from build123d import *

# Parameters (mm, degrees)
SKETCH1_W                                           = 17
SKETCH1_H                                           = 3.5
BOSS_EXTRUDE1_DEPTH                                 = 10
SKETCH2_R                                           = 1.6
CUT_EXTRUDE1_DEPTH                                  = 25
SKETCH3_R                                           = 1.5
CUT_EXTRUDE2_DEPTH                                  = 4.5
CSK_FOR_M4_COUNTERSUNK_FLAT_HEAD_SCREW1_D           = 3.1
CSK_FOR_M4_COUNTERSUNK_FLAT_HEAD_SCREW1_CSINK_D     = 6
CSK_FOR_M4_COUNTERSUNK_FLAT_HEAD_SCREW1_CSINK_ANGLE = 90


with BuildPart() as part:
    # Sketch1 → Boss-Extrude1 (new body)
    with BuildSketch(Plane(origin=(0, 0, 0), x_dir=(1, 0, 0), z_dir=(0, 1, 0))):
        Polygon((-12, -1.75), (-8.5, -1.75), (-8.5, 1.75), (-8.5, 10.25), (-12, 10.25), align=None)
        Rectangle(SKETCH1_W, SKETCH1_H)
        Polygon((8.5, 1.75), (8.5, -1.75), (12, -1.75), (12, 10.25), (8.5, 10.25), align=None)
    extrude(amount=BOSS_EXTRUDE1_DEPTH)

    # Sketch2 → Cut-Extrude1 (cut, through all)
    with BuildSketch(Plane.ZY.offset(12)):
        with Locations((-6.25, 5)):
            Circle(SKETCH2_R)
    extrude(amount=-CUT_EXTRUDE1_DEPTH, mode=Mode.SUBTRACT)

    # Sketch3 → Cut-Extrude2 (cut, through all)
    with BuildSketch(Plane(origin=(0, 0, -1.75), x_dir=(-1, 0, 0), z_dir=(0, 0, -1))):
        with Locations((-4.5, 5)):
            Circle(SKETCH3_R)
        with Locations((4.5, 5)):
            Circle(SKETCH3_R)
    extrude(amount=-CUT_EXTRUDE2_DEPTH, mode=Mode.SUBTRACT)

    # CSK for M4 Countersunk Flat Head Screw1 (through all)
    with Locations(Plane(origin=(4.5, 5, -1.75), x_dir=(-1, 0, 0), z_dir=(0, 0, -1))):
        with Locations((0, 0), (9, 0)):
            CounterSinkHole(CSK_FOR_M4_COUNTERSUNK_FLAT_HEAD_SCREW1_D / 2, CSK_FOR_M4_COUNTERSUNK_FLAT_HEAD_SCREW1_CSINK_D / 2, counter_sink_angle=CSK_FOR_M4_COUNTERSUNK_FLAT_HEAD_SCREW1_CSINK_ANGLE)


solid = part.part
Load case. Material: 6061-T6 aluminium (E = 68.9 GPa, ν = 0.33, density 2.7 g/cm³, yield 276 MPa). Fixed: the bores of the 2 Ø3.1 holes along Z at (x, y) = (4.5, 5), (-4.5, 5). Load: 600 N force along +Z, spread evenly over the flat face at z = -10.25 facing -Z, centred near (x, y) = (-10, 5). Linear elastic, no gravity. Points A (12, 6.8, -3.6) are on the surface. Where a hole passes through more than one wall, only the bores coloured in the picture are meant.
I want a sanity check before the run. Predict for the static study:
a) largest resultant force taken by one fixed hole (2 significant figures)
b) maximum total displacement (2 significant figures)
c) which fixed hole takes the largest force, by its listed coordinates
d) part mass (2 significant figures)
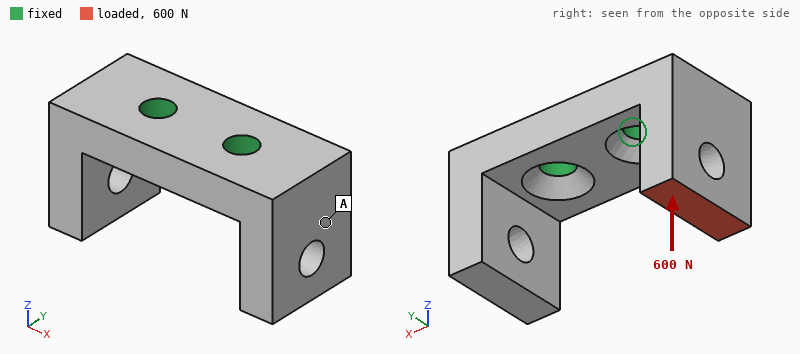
750 N
74 µm
(-4.5, 5)
3.5 g
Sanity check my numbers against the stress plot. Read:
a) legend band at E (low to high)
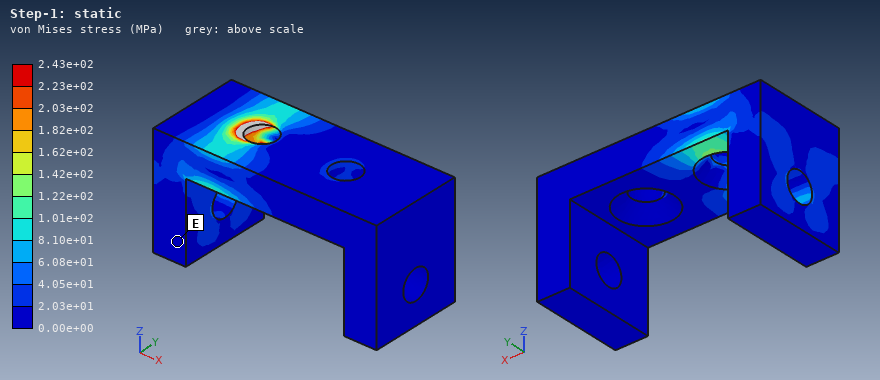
0.00e+00 to 2.03e+01 MPa
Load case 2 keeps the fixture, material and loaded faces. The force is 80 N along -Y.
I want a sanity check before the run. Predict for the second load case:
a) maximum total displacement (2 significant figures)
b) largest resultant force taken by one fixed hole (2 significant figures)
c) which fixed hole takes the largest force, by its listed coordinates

23 µm
97 N
(-4.5, 5)
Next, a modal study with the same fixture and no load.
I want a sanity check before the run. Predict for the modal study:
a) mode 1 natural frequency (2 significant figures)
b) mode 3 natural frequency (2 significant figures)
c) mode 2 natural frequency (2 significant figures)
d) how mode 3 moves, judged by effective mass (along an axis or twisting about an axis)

13 kHz
16 kHz
13 kHz
along Y
